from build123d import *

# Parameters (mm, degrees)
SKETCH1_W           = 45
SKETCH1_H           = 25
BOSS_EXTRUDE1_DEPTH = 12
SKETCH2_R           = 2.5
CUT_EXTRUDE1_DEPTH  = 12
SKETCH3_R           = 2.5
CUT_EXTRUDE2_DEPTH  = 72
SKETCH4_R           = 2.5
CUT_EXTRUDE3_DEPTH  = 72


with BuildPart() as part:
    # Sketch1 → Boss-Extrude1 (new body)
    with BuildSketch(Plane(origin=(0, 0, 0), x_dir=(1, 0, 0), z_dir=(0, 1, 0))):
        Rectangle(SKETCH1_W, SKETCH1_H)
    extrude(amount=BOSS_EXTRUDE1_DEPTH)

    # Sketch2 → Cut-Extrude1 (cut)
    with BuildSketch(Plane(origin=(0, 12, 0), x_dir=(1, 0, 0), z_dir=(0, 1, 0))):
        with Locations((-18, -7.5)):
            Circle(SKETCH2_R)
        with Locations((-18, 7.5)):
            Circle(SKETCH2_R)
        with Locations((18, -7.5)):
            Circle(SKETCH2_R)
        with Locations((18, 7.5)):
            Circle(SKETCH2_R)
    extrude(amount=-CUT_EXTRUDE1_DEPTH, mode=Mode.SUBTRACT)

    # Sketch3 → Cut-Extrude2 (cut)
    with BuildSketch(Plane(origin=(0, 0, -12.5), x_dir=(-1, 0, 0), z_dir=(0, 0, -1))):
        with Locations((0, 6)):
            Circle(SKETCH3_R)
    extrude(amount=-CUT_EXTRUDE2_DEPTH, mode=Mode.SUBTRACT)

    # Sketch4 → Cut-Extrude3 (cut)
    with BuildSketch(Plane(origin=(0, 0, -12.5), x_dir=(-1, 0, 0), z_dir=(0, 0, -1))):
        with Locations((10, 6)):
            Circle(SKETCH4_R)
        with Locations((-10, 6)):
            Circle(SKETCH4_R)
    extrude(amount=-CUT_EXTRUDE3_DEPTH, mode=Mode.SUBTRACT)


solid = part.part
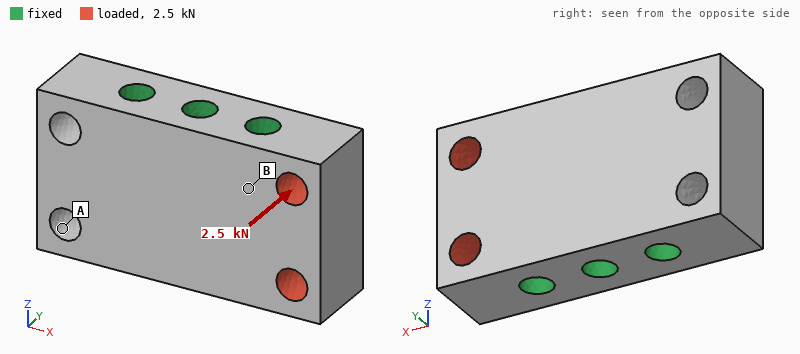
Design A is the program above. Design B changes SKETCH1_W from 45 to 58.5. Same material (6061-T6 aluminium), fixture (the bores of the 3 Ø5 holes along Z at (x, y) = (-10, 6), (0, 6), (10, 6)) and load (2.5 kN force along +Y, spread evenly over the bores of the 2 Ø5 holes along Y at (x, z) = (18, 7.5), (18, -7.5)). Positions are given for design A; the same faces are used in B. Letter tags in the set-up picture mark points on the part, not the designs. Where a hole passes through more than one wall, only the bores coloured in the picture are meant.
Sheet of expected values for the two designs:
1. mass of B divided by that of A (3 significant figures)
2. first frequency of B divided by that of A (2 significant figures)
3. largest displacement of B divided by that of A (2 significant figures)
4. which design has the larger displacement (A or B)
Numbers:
1.37
0.46
1.3
B
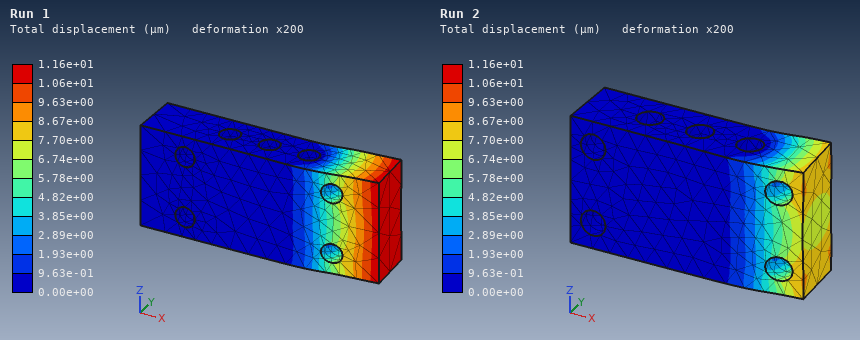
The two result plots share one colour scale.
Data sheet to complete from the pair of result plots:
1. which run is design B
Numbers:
Run 1
